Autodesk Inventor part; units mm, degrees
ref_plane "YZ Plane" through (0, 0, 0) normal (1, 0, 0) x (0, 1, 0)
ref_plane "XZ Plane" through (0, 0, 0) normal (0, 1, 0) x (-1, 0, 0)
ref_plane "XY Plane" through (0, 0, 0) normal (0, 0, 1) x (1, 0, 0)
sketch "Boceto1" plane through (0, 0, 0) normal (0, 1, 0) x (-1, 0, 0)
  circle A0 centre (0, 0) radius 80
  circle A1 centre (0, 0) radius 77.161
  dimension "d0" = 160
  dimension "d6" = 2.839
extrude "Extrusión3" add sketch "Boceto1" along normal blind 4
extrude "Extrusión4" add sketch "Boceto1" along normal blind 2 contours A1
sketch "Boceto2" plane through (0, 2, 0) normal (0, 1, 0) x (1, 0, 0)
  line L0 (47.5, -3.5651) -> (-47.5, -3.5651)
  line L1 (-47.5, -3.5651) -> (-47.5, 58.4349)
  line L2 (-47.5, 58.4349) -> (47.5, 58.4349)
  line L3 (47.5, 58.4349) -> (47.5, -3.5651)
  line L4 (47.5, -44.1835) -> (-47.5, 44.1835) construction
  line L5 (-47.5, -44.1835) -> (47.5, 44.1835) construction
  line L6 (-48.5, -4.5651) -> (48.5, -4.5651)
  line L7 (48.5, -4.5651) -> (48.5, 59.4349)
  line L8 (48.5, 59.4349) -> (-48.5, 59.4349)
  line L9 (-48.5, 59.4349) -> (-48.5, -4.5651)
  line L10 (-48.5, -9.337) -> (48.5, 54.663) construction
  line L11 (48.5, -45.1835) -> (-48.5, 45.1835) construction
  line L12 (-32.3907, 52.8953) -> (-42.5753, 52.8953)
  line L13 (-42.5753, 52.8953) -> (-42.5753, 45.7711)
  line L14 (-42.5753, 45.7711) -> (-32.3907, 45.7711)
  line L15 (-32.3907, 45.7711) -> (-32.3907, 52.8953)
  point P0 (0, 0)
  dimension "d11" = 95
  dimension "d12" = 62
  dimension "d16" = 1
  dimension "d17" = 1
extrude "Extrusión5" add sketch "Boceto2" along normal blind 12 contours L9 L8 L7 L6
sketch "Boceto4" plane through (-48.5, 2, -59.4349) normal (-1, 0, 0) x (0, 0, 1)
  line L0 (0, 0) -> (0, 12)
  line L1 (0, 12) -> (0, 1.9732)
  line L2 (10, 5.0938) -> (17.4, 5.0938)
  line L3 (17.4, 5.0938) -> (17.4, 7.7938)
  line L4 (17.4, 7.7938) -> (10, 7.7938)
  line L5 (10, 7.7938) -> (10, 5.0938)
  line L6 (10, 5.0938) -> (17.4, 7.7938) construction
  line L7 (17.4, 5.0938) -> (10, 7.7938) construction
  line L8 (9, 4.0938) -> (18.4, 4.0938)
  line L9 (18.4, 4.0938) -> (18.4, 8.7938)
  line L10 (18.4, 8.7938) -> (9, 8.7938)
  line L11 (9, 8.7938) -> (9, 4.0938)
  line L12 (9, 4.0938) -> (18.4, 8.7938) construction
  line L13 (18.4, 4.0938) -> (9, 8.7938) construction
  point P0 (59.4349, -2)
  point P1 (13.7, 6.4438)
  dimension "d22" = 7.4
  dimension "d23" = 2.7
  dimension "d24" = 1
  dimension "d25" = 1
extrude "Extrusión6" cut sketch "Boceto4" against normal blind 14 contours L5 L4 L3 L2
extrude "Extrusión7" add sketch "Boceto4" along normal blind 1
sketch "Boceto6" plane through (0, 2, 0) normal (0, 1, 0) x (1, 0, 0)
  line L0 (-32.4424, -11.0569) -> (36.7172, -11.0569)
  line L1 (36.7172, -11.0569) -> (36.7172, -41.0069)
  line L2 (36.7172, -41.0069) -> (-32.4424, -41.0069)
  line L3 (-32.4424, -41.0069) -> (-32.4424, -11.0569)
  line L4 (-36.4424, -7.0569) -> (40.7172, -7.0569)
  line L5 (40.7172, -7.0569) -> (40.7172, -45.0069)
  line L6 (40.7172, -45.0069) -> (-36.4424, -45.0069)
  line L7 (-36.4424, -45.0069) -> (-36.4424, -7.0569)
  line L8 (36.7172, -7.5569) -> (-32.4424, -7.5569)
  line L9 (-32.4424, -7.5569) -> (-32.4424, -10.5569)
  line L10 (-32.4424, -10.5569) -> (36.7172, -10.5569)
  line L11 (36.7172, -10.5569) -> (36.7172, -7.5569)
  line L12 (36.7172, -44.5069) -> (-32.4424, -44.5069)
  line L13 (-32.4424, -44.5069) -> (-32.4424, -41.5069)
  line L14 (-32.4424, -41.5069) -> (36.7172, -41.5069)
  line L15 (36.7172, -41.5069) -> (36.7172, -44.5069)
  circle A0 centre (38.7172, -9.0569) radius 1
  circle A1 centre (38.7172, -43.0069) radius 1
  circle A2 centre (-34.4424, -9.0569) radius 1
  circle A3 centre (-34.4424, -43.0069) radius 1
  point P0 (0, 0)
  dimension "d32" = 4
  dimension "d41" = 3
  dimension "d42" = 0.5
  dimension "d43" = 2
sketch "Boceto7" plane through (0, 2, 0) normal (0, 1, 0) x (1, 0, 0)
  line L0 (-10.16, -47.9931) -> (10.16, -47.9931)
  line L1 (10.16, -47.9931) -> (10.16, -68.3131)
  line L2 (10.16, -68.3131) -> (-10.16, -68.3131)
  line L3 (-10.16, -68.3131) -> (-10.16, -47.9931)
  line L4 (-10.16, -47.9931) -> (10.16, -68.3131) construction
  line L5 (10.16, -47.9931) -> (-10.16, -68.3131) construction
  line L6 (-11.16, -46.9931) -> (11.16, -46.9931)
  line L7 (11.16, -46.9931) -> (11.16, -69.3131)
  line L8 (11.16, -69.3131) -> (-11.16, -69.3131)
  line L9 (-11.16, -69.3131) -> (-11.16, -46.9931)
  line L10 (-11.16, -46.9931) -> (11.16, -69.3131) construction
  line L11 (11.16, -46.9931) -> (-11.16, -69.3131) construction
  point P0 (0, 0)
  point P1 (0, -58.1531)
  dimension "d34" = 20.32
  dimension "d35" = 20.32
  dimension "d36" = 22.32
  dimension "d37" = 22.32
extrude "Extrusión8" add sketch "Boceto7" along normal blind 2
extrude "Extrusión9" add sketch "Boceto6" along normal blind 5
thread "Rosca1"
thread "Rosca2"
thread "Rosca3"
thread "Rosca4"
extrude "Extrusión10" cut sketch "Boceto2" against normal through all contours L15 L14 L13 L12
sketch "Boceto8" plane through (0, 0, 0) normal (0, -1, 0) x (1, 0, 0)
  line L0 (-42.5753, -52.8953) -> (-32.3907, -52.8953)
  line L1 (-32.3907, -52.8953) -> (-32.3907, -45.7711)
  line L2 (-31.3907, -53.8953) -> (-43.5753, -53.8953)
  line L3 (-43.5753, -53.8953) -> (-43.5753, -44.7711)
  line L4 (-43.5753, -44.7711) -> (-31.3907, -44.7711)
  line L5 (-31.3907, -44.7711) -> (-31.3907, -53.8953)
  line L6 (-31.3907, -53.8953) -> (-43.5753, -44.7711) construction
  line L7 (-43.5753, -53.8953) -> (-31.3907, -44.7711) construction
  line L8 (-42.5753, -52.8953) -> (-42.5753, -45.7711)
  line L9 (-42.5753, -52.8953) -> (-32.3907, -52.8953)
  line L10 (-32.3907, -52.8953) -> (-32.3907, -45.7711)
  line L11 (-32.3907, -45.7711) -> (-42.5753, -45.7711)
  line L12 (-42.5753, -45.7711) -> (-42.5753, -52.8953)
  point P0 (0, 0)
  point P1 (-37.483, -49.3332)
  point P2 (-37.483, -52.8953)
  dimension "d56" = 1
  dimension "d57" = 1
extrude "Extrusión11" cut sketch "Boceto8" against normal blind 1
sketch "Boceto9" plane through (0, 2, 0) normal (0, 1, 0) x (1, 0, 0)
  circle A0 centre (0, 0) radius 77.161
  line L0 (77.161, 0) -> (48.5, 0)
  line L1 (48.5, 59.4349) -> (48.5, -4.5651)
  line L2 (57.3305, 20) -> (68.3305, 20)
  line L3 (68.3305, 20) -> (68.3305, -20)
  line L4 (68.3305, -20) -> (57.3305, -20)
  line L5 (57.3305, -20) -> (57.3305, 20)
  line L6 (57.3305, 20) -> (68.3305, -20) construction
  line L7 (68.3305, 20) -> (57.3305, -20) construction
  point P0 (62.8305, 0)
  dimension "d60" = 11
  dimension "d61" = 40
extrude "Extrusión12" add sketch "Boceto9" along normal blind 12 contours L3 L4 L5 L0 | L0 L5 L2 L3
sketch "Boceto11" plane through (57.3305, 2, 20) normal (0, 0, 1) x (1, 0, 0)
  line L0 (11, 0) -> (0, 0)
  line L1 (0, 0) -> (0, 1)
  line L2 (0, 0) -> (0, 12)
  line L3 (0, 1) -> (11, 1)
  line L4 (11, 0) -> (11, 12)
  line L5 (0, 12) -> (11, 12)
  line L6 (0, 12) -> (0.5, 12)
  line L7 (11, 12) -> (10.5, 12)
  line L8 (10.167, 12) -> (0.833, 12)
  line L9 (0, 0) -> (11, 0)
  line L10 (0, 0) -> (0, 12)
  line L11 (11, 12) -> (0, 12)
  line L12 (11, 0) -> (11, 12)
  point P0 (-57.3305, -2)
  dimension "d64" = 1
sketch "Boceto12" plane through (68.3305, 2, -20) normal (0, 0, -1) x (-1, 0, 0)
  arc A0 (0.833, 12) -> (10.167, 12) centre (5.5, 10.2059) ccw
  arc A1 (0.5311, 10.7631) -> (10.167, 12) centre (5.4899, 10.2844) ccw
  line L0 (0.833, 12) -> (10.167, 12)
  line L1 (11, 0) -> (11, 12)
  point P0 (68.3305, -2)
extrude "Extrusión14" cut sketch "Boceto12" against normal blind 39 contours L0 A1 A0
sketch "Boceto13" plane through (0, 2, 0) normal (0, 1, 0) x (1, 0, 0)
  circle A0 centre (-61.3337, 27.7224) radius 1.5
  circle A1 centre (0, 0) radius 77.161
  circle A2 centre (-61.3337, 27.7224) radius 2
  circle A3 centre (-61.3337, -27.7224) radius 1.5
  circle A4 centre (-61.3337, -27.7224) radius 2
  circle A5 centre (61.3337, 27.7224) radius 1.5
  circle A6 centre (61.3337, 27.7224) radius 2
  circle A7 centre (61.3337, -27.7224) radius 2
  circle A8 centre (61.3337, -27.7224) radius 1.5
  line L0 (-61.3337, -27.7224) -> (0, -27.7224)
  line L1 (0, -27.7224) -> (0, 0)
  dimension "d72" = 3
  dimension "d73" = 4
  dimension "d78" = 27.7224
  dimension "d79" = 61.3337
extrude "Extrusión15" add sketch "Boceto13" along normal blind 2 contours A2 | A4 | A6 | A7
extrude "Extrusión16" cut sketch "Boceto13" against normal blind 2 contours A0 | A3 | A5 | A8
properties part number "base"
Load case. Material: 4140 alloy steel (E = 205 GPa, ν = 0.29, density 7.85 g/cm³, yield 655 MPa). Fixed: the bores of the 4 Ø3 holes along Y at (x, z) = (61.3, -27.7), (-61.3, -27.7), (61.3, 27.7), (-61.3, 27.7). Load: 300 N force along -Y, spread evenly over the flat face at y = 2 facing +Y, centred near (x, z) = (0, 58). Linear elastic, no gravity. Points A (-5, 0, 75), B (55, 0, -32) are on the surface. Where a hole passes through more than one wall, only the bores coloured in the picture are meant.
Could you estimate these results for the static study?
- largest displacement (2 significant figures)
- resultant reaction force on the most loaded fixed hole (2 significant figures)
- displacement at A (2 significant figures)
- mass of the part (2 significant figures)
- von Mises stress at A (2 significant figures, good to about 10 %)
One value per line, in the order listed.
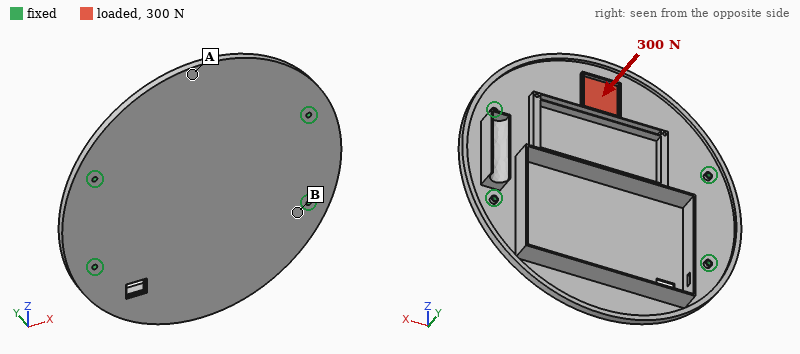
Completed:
0.53 mm
270 N
0.49 mm
410 g
56 MPa
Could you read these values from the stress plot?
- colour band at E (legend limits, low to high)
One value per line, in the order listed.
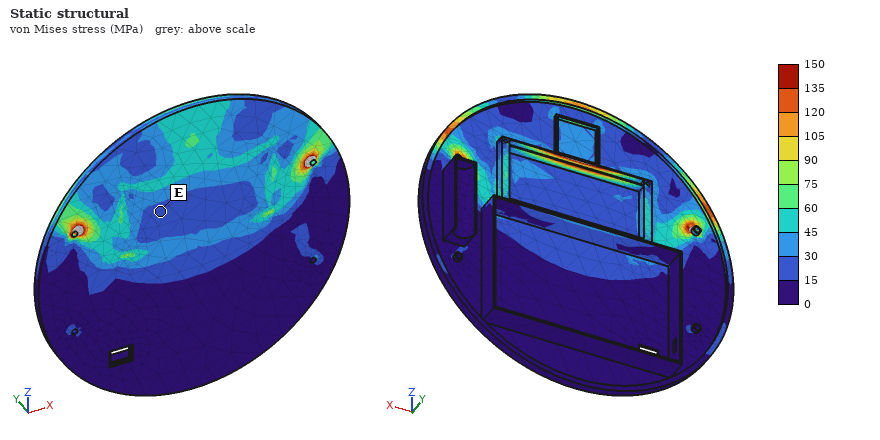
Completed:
15 to 30 MPa
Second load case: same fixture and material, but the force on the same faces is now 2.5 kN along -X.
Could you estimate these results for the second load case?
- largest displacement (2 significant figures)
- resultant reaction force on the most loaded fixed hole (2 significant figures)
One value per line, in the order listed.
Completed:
30 µm
1.2 kN
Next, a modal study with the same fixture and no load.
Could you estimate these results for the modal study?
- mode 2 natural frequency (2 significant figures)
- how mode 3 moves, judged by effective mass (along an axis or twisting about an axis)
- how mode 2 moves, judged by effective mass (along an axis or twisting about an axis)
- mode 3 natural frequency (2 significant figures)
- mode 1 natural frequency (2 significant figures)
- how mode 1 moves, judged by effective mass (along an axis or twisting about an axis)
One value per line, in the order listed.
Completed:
910 Hz
along Y
along Y
1200 Hz
610 Hz
along Y
